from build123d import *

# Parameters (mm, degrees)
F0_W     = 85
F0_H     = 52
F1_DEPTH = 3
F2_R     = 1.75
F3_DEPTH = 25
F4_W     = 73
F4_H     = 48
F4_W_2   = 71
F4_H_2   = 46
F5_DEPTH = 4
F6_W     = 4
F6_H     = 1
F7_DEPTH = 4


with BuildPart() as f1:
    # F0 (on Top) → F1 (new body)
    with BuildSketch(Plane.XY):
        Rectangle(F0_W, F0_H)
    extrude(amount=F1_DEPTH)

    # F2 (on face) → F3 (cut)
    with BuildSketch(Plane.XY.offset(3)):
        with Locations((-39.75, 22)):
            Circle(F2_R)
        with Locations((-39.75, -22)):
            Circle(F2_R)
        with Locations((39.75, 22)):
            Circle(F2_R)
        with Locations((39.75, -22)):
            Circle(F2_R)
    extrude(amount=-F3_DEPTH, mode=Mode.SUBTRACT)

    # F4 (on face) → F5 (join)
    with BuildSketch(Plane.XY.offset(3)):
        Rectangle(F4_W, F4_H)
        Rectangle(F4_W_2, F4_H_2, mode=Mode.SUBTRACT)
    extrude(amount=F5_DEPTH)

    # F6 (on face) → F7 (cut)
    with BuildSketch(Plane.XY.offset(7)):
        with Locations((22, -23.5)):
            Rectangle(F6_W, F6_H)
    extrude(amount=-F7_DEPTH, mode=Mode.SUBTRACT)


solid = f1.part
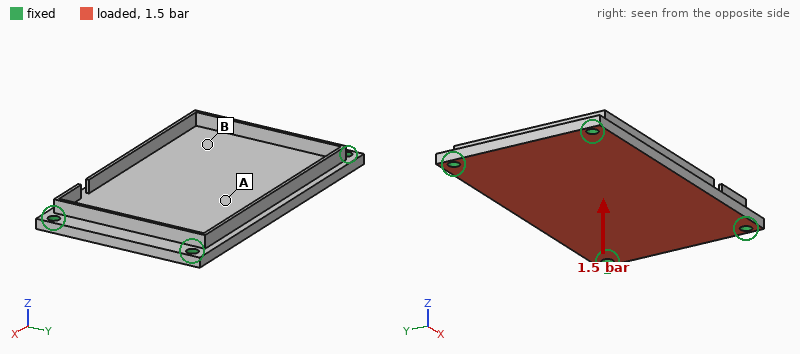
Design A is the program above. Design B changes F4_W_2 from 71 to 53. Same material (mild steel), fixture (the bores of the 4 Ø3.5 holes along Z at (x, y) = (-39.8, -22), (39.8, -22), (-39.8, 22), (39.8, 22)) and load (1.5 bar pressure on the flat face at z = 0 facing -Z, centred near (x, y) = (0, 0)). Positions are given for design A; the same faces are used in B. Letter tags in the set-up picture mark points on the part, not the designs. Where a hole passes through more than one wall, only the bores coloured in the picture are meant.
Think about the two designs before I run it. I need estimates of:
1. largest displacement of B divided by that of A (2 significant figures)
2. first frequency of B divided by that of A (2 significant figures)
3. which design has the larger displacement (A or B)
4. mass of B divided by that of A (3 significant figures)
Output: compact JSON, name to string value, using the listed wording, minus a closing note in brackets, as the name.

{"largest displacement of B divided by that of A": "0.88", "first frequency of B divided by that of A": "1.0", "which design has the larger displacement": "A", "mass of B divided by that of A": "1.24"}
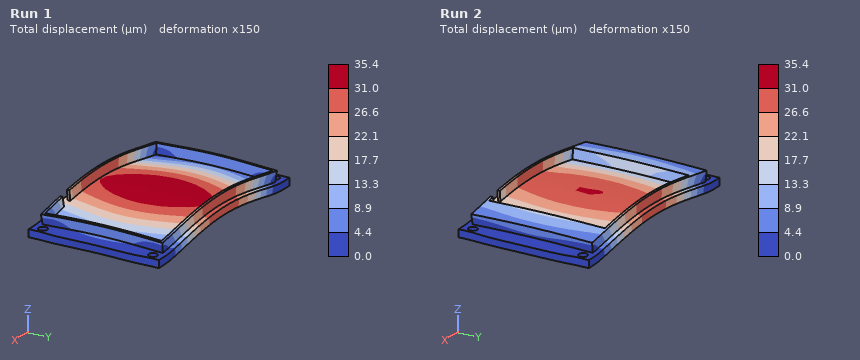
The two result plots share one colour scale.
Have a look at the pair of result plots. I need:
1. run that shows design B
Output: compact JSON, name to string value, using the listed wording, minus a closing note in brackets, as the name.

{"run that shows design B": "Run 2"}
